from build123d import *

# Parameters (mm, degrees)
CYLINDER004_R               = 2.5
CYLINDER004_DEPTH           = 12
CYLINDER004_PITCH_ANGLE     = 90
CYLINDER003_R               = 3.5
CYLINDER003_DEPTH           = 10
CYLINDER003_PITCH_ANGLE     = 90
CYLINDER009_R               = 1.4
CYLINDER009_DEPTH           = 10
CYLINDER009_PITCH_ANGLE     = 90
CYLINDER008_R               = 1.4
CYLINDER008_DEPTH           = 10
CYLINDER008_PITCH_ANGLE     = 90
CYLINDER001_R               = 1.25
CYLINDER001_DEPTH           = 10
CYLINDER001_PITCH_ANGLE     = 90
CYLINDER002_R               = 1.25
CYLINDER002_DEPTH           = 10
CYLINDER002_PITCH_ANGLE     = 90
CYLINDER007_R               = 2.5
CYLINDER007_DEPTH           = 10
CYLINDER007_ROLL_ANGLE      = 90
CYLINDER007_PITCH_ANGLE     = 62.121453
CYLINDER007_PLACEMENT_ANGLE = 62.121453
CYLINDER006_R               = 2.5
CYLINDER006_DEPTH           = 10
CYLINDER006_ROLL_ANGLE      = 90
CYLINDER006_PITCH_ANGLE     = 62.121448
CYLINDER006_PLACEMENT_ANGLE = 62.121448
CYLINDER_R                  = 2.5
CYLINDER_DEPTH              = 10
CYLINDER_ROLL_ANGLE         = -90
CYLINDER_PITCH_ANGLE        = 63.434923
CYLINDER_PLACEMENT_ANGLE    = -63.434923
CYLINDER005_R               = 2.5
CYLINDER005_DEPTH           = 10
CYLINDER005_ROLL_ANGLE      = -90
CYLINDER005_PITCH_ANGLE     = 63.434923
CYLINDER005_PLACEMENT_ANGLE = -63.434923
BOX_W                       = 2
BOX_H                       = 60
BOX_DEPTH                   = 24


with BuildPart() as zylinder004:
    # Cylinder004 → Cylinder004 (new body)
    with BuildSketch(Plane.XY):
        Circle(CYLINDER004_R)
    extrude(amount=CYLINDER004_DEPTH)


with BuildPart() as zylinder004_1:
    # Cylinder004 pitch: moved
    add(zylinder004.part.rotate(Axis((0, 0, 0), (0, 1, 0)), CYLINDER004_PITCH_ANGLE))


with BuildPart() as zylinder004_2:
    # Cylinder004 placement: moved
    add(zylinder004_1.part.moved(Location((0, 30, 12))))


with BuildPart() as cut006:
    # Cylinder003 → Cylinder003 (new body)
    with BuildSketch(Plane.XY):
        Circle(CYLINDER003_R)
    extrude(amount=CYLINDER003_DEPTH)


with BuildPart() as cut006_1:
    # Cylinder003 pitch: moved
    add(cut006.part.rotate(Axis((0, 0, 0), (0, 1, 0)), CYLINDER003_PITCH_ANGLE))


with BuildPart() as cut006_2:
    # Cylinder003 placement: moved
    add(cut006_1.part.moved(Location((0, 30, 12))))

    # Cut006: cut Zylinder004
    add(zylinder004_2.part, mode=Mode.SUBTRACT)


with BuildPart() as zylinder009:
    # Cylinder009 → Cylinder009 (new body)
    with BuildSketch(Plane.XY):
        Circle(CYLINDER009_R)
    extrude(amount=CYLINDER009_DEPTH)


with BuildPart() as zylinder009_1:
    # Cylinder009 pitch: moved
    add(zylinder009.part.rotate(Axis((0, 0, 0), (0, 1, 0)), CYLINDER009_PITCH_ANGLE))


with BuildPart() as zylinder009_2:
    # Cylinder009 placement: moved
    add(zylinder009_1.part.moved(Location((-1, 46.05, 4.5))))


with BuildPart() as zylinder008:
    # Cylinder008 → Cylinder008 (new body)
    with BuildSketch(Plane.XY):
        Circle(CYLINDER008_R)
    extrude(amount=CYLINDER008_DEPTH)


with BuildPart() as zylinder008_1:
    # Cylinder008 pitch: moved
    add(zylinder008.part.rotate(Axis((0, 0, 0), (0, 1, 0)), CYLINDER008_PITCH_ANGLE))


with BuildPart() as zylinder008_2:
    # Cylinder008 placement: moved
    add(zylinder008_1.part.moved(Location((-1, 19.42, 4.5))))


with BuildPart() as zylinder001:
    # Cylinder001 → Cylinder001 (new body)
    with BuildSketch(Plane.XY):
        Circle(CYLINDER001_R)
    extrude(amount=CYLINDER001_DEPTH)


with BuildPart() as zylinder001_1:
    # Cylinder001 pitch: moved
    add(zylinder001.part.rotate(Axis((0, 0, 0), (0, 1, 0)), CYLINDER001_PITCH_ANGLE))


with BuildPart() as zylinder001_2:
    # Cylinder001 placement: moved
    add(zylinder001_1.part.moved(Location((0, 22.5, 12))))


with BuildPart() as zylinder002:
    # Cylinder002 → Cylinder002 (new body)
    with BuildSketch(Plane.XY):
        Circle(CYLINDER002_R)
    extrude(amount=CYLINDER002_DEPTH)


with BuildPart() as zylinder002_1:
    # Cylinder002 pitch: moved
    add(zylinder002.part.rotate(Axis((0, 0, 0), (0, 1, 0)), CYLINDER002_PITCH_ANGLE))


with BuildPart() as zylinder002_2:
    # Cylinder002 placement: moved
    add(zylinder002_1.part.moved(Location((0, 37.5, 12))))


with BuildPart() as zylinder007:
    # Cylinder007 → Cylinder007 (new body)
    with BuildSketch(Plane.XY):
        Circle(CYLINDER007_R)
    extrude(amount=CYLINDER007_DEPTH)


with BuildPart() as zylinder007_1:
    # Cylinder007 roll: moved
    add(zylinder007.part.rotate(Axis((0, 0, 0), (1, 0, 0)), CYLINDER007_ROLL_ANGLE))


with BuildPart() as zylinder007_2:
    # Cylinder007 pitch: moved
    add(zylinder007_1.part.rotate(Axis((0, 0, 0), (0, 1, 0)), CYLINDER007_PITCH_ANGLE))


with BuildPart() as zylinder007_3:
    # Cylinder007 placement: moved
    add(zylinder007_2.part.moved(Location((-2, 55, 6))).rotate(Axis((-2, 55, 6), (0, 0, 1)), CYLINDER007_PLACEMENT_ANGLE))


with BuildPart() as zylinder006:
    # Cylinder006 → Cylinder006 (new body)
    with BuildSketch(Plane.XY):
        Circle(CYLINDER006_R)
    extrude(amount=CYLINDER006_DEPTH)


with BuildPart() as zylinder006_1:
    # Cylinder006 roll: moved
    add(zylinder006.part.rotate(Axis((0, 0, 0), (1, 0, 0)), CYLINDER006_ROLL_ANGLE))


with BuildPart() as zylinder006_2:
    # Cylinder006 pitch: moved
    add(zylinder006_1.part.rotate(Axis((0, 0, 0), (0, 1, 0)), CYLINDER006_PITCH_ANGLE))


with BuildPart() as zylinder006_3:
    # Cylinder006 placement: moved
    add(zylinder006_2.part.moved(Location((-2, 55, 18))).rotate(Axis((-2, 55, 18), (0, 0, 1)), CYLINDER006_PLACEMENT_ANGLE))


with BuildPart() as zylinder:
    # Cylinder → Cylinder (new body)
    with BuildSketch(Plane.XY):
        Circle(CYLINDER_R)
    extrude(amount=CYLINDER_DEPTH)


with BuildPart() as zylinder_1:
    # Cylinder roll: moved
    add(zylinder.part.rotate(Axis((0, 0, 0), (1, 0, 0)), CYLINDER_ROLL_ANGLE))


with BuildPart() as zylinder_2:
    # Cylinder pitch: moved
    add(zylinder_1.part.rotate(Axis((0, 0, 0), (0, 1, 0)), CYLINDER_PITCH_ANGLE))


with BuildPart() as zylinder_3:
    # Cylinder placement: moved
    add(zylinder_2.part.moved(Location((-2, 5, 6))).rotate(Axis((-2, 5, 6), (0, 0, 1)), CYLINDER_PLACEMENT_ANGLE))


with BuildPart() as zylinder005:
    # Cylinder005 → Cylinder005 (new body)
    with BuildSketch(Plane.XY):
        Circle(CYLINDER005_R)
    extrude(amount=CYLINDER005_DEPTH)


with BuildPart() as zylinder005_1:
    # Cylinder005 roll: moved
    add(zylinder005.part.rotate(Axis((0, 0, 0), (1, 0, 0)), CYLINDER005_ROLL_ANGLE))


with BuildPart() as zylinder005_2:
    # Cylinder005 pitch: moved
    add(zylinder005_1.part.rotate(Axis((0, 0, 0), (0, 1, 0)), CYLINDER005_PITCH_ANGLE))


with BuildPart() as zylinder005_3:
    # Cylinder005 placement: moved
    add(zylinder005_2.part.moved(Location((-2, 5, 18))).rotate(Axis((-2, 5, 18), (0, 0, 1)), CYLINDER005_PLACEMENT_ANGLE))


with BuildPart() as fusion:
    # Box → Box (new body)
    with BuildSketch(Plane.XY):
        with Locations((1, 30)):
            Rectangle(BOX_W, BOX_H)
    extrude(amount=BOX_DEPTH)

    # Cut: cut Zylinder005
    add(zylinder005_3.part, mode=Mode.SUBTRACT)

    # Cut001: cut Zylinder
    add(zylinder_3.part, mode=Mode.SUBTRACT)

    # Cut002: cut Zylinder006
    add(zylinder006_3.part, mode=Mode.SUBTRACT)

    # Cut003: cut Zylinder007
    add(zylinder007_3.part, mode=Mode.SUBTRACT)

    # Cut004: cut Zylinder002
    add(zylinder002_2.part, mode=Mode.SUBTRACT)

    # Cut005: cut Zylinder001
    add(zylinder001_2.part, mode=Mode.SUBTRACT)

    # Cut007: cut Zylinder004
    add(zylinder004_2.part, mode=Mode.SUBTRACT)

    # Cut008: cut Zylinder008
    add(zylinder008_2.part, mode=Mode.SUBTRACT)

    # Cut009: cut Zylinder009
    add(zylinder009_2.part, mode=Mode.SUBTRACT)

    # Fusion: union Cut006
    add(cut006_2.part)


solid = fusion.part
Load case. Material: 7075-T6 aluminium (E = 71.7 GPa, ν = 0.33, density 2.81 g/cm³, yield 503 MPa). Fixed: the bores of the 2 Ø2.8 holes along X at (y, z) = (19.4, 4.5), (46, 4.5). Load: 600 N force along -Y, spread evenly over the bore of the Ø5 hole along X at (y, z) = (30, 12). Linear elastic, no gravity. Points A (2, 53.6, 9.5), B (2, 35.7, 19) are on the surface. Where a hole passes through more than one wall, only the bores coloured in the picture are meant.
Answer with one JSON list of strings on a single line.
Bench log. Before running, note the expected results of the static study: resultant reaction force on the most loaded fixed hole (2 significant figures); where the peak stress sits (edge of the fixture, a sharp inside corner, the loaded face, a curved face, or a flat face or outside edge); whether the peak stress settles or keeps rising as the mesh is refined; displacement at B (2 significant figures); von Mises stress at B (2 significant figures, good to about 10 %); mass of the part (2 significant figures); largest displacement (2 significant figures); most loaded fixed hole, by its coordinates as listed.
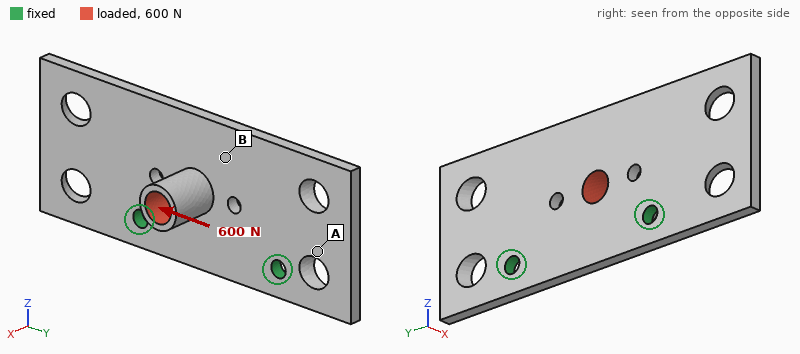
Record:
["380 N", "edge of the fixture", "keeps rising", "30 µm", "44 MPa", "7.8 g", "73 µm", "(19.4, 4.5)"]
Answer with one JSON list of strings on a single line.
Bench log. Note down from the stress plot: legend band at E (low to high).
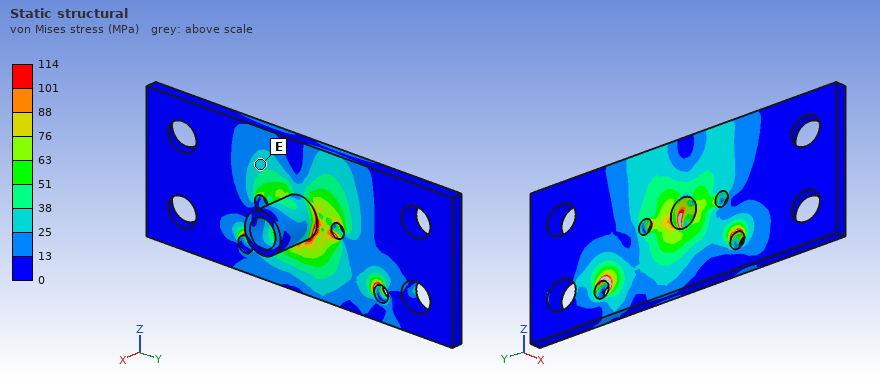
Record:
["25 to 38 MPa"]
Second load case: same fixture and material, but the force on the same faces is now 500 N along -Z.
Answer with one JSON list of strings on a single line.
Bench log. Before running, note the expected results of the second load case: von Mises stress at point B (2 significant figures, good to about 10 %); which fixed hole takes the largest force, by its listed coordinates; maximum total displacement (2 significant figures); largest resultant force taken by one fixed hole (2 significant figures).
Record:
["21 MPa", "(19.4, 4.5)", "0.16 mm", "320 N"]
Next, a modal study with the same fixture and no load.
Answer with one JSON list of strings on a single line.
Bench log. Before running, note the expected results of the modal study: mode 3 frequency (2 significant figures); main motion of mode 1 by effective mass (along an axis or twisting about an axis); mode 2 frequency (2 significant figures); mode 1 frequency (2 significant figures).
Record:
["4900 Hz", "along X", "3700 Hz", "3200 Hz"]
